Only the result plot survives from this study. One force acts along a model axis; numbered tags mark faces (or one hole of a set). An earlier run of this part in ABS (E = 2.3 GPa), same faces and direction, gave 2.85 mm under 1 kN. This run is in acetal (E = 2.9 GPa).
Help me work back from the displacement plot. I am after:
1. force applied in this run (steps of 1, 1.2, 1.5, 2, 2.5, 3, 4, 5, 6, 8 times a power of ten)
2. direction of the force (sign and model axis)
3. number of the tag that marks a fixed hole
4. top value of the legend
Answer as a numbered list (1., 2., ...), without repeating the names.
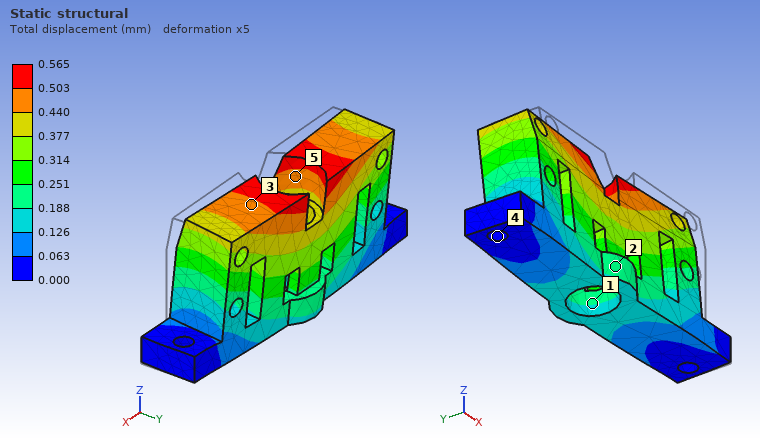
1. 250 N
2. +Y
3. 4
4. 0.565 mm
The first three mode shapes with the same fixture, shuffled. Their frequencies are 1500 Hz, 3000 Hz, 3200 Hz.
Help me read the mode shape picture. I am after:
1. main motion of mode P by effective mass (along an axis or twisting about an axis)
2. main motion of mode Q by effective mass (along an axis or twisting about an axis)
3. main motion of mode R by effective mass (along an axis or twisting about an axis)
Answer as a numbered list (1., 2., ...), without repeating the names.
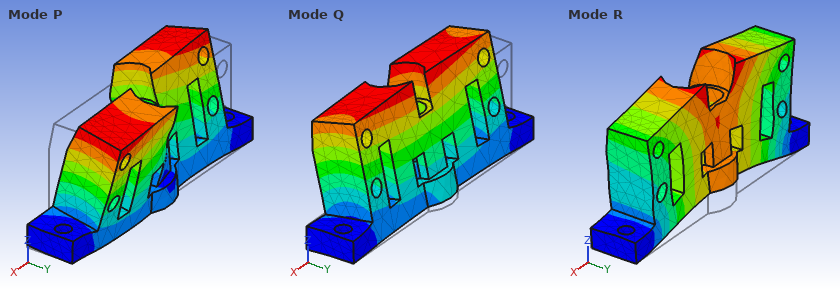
1. twisting about Z
2. along Y
3. along Z
